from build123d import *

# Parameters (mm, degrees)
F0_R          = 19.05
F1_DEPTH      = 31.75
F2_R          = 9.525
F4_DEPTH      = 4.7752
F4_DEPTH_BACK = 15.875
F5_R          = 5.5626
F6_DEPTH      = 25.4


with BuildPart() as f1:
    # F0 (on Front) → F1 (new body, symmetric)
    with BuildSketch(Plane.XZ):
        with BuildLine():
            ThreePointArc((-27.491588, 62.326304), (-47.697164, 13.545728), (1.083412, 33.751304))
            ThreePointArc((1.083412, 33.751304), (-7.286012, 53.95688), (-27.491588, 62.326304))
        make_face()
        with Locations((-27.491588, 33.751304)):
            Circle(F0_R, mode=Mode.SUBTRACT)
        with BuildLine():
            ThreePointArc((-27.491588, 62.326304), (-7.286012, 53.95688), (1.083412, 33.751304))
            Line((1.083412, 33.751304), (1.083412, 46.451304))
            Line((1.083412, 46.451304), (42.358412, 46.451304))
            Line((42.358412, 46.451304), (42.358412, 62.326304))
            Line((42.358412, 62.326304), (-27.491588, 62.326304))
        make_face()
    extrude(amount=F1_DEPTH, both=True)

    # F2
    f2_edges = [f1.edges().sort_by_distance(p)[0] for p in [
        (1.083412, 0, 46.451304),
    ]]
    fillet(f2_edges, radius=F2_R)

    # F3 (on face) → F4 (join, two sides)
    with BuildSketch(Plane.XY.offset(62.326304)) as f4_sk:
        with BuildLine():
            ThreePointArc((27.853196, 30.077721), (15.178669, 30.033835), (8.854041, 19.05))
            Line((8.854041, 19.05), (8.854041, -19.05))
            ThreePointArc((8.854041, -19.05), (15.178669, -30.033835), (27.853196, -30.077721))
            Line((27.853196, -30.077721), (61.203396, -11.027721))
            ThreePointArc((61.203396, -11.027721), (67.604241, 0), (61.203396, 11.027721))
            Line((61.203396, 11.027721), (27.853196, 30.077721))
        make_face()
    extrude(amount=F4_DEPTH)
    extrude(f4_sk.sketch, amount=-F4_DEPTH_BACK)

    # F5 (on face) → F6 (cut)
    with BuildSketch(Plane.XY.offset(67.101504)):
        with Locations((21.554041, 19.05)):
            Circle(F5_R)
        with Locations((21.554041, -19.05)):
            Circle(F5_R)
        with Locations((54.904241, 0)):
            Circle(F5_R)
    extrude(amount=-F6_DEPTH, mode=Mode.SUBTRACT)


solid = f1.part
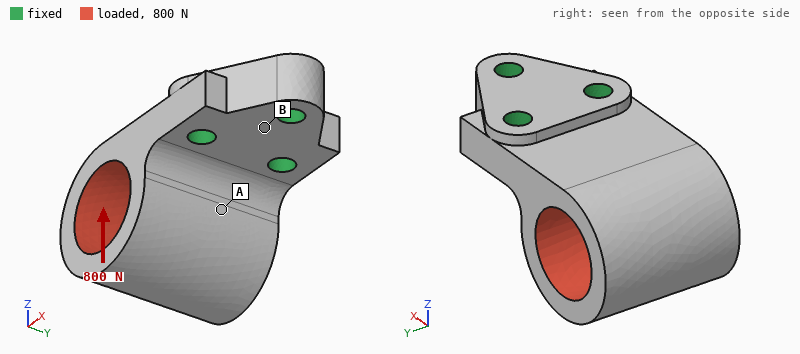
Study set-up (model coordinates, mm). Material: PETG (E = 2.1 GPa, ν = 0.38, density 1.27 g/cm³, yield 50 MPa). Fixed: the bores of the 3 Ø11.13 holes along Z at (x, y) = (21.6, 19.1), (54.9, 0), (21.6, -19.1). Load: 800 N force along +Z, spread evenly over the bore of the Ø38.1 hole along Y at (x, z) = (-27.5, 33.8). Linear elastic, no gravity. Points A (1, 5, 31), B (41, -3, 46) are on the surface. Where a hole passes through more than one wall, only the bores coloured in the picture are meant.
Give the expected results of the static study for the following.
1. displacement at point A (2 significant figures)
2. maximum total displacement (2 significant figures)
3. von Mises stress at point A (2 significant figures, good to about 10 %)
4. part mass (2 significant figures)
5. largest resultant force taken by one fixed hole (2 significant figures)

0.28 mm
1.0 mm
2.5 MPa
210 g
470 N
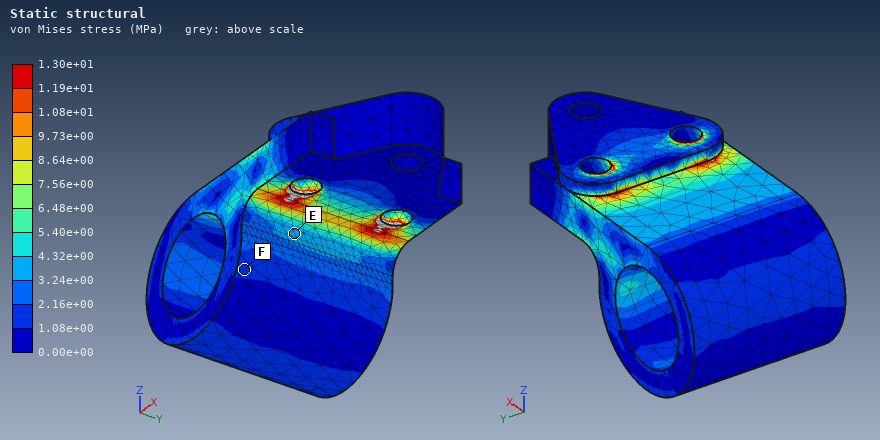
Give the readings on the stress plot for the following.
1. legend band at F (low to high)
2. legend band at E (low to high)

1.08e+00 to 2.16e+00 MPa
3.24e+00 to 4.32e+00 MPa
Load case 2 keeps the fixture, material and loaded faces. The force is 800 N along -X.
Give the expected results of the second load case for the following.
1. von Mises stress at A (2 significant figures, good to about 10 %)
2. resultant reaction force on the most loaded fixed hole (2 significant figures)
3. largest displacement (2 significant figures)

2.5 MPa
380 N
0.63 mm
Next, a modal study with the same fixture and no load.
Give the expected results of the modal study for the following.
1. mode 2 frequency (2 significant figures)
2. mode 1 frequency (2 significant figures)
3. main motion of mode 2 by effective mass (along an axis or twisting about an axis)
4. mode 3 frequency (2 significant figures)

980 Hz
430 Hz
along Y
1600 Hz
